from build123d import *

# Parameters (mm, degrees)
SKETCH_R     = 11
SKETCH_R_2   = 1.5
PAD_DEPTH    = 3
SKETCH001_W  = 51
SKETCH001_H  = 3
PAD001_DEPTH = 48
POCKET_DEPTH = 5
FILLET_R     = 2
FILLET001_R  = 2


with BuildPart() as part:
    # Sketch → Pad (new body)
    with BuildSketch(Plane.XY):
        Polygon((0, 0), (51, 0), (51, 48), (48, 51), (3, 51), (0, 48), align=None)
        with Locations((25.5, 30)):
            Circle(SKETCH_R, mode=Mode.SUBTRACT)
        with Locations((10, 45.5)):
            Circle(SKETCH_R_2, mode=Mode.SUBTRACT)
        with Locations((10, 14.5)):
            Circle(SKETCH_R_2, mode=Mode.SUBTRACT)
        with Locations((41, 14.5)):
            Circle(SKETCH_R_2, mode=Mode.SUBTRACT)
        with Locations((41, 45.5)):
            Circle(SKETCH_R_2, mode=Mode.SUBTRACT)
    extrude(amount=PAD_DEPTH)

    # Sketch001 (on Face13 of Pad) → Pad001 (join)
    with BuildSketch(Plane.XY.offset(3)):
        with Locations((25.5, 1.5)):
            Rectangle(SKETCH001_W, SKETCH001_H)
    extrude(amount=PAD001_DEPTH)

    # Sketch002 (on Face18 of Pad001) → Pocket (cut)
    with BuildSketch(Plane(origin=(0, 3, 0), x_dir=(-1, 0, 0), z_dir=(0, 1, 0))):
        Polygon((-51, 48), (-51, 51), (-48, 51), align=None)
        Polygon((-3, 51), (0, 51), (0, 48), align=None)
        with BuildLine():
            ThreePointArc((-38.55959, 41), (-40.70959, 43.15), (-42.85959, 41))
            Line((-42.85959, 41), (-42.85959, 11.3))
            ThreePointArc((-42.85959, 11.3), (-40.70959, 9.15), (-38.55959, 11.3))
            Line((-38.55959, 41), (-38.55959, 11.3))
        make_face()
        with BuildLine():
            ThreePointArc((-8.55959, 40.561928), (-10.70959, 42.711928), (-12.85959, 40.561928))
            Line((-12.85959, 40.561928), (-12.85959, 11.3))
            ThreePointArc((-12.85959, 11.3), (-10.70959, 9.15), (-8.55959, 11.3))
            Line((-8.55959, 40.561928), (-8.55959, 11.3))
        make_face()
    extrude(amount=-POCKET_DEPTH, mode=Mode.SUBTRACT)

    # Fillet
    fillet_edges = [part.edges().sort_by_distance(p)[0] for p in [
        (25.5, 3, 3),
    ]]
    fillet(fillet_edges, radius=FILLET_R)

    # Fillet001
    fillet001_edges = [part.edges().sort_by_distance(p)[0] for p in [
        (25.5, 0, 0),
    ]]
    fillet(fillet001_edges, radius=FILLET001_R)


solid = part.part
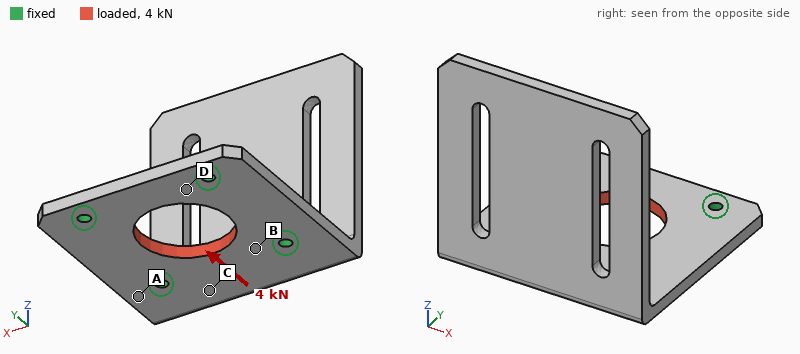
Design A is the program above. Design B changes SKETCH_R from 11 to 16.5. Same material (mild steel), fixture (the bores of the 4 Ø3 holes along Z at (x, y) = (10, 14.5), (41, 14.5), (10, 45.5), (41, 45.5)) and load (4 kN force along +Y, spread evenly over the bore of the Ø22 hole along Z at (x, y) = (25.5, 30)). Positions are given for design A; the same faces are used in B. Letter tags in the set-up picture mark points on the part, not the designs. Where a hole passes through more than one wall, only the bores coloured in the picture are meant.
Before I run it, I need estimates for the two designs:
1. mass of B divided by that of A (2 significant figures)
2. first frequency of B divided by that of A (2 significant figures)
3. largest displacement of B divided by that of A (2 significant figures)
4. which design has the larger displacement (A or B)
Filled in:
0.89
0.97
1.8
B
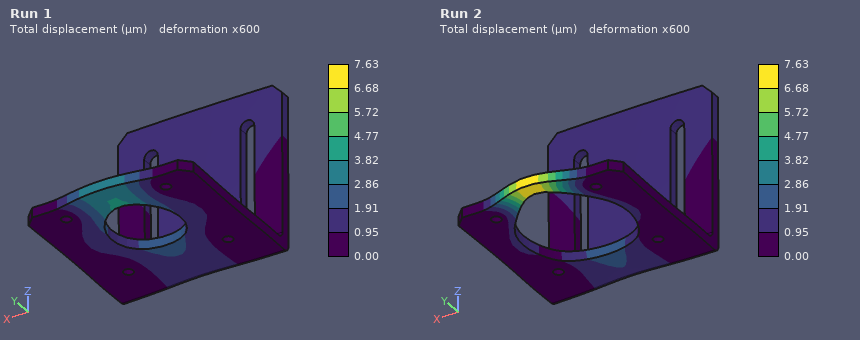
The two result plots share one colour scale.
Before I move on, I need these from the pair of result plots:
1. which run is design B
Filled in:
Run 2
